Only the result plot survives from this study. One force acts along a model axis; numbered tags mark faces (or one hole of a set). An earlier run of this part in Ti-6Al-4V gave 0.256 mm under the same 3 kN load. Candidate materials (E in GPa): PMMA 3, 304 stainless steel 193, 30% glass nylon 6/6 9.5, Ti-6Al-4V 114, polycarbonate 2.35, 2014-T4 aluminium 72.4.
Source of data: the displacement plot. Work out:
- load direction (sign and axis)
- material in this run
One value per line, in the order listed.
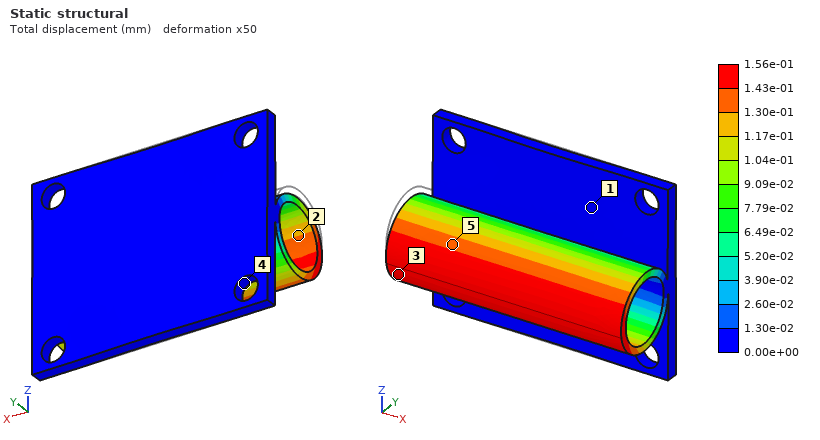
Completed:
-Z
304 stainless steel
